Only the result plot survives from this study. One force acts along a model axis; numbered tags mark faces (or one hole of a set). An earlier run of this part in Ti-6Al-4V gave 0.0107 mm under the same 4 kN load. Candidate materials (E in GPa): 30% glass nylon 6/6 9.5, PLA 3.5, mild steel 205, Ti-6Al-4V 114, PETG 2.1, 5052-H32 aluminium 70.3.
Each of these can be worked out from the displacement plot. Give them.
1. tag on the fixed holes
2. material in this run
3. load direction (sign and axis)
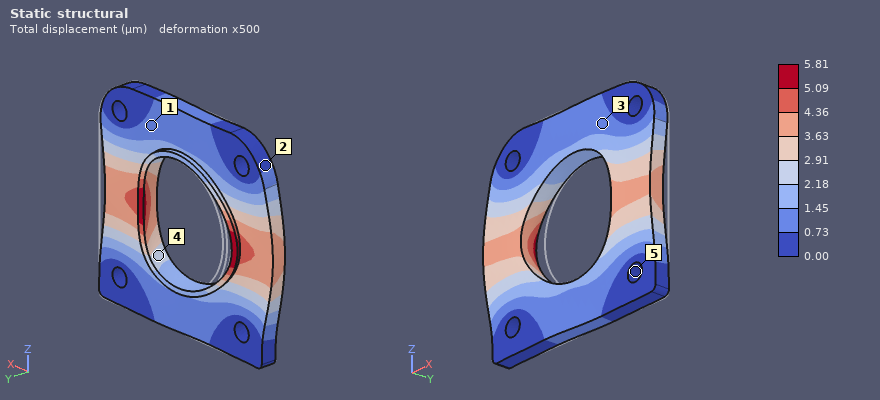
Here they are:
5
mild steel
-X
